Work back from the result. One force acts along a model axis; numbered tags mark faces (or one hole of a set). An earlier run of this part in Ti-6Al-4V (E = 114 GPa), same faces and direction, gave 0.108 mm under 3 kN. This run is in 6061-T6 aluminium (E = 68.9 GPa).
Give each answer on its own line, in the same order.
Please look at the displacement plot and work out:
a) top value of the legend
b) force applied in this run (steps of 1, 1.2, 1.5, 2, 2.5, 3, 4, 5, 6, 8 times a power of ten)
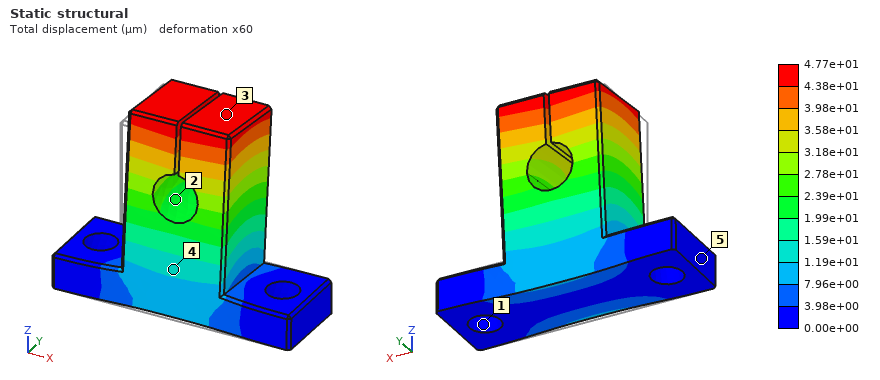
4.77e+01 µm
800 N
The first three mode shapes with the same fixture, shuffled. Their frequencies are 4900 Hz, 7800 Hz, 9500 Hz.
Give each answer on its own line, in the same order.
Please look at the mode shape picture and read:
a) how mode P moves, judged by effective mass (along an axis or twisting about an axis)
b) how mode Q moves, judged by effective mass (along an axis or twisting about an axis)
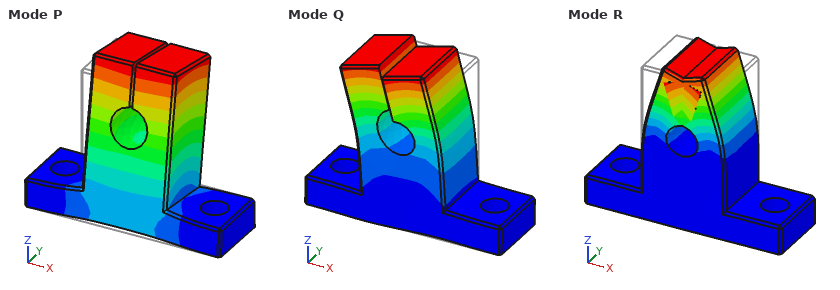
along Y
along X
